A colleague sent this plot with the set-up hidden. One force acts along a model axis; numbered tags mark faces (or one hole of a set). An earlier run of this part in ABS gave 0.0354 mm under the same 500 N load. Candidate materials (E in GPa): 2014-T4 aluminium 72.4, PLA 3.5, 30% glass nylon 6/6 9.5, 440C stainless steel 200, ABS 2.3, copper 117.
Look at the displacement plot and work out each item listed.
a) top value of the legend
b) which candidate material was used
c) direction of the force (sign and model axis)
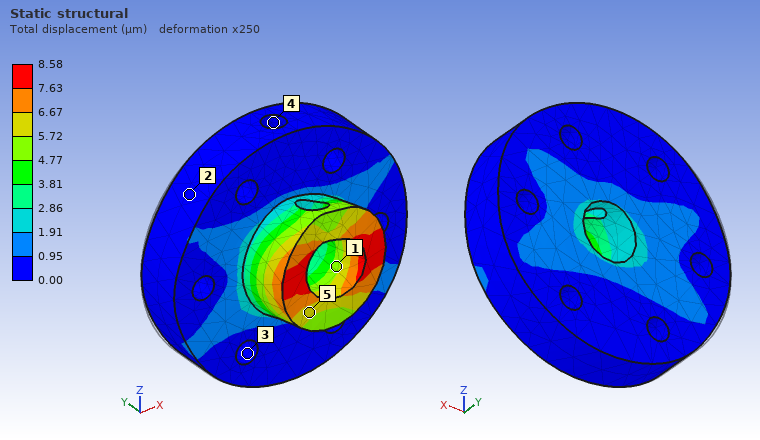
8.58 µm
30% glass nylon 6/6
+X
